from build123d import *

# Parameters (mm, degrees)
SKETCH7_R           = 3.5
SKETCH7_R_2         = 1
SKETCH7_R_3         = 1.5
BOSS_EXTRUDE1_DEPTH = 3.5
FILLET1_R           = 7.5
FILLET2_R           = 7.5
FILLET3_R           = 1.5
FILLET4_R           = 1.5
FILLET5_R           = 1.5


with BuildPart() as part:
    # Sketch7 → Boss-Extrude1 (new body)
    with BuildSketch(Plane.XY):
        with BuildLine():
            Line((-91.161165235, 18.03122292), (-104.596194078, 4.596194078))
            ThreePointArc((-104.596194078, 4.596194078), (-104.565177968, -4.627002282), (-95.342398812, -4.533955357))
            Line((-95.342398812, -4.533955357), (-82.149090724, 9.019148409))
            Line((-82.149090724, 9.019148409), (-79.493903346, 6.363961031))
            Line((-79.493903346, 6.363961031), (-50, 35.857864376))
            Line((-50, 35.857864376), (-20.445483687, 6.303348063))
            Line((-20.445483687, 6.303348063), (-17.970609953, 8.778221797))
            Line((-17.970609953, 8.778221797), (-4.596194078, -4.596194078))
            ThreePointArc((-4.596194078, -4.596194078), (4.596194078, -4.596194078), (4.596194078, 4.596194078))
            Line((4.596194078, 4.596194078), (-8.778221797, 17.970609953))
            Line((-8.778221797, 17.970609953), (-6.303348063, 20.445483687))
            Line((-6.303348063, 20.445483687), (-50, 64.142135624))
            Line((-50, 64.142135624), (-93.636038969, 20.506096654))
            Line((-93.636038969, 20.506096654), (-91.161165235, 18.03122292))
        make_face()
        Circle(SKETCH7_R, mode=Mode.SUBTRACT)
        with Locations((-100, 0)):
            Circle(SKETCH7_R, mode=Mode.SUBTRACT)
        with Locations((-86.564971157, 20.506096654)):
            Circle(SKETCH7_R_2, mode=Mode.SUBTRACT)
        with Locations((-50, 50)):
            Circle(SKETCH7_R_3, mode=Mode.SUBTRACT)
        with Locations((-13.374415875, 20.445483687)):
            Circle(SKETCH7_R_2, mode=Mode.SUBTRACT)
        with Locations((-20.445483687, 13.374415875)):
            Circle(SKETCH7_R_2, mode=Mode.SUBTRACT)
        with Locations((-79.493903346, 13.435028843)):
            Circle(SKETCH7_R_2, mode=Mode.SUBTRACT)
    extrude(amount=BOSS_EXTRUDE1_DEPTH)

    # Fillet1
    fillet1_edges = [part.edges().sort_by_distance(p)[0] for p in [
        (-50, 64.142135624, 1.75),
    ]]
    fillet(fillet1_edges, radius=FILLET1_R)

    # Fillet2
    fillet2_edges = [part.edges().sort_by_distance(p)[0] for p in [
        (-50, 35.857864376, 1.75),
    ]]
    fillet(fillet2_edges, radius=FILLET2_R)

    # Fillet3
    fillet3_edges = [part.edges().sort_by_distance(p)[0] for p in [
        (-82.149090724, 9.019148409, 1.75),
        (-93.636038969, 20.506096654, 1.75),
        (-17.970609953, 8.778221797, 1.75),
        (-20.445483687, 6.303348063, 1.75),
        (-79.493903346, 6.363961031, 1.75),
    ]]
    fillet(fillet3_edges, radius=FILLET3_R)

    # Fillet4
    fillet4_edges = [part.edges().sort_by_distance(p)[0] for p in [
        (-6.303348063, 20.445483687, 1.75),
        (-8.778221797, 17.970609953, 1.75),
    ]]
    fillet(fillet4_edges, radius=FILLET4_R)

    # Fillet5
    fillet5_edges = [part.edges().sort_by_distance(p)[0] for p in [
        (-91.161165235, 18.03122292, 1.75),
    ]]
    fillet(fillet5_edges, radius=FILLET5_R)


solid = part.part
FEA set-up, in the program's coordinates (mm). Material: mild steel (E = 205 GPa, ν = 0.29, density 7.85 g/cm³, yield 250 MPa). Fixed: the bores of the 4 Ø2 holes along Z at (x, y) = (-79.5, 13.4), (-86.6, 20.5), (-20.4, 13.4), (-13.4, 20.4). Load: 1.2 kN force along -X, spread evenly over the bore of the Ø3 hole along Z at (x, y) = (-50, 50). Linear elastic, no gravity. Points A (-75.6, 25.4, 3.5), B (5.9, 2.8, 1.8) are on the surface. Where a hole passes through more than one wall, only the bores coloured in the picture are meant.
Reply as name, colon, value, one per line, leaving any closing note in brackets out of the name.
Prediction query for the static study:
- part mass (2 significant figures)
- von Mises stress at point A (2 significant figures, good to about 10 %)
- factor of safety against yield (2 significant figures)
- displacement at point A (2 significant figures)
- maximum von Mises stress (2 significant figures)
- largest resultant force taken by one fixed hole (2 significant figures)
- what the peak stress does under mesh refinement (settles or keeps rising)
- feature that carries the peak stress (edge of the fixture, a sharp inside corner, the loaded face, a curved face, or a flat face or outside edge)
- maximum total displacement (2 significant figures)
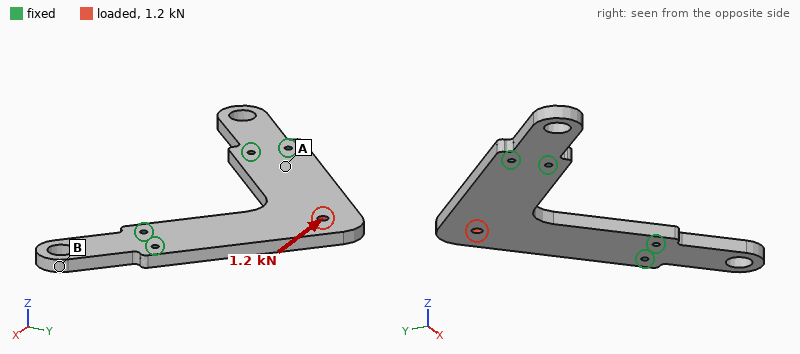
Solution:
part mass: 71 g
von Mises stress at point A: 13 MPa
factor of safety against yield: 3.9
displacement at point A: 0.85 µm
maximum von Mises stress: 65 MPa
largest resultant force taken by one fixed hole: 530 N
what the peak stress does under mesh refinement: settles
feature that carries the peak stress: the loaded face
maximum total displacement: 4.9 µm
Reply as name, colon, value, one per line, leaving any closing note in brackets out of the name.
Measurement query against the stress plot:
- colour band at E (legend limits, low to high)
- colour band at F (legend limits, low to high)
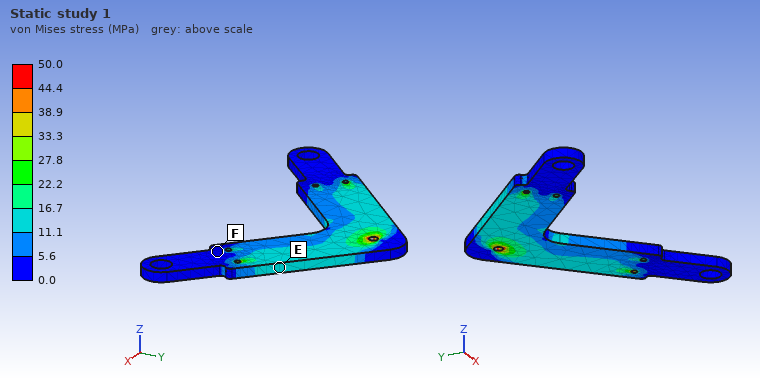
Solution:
colour band at E: 11.1 to 16.7 MPa
colour band at F: 0.0 to 5.6 MPa
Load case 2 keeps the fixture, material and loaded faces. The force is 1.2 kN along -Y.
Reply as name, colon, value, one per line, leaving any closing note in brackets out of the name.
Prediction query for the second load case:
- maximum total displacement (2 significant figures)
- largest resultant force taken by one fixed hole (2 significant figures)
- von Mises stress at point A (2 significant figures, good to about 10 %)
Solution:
maximum total displacement: 4.3 µm
largest resultant force taken by one fixed hole: 550 N
von Mises stress at point A: 12 MPa
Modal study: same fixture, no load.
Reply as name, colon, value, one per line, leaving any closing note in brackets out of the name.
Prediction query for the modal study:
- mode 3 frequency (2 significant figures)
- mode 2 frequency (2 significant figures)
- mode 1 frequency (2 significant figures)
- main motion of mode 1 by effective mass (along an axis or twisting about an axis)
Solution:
mode 3 frequency: 4000 Hz
mode 2 frequency: 4000 Hz
mode 1 frequency: 1600 Hz
main motion of mode 1 by effective mass: along Z
